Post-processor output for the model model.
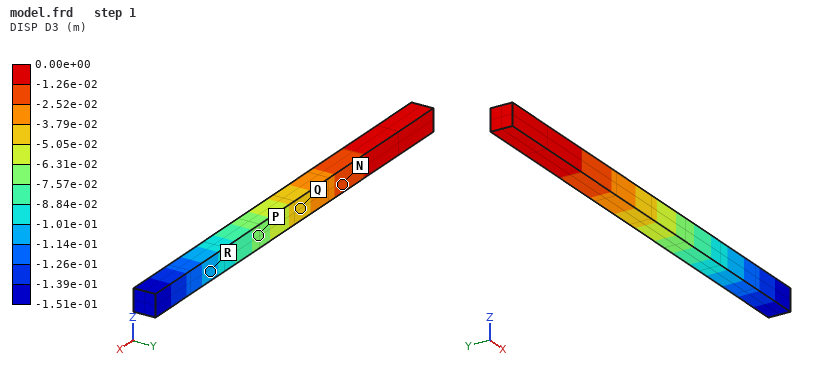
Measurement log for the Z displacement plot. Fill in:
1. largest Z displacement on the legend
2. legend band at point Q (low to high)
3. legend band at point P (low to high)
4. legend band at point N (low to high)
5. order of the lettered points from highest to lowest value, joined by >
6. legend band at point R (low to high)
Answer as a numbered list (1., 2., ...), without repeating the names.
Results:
1. 0.00e+00 m
2. -5.05e-02 to -3.79e-02 m
3. -7.57e-02 to -6.31e-02 m
4. -2.52e-02 to -1.26e-02 m
5. N > Q > P > R
6. -1.14e-01 to -1.01e-01 m
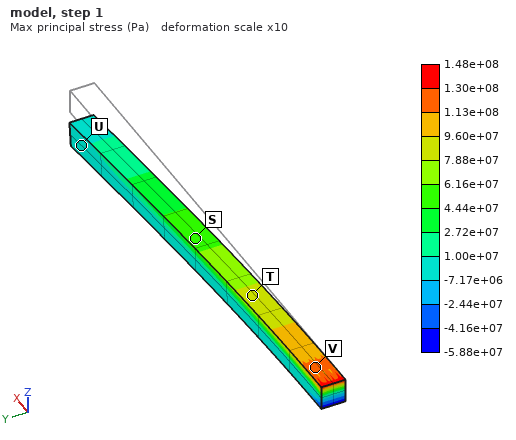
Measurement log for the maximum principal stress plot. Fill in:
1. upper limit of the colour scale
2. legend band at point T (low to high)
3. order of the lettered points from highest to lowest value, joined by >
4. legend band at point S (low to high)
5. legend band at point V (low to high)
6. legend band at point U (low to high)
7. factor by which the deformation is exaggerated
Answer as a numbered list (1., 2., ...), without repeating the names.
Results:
1. 1.48e+08 Pa
2. 7.88e+07 to 9.60e+07 Pa
3. V > T > S > U
4. 4.44e+07 to 6.16e+07 Pa
5. 1.13e+08 to 1.30e+08 Pa
6. -7.17e+06 to 1.00e+07 Pa
7. 10
